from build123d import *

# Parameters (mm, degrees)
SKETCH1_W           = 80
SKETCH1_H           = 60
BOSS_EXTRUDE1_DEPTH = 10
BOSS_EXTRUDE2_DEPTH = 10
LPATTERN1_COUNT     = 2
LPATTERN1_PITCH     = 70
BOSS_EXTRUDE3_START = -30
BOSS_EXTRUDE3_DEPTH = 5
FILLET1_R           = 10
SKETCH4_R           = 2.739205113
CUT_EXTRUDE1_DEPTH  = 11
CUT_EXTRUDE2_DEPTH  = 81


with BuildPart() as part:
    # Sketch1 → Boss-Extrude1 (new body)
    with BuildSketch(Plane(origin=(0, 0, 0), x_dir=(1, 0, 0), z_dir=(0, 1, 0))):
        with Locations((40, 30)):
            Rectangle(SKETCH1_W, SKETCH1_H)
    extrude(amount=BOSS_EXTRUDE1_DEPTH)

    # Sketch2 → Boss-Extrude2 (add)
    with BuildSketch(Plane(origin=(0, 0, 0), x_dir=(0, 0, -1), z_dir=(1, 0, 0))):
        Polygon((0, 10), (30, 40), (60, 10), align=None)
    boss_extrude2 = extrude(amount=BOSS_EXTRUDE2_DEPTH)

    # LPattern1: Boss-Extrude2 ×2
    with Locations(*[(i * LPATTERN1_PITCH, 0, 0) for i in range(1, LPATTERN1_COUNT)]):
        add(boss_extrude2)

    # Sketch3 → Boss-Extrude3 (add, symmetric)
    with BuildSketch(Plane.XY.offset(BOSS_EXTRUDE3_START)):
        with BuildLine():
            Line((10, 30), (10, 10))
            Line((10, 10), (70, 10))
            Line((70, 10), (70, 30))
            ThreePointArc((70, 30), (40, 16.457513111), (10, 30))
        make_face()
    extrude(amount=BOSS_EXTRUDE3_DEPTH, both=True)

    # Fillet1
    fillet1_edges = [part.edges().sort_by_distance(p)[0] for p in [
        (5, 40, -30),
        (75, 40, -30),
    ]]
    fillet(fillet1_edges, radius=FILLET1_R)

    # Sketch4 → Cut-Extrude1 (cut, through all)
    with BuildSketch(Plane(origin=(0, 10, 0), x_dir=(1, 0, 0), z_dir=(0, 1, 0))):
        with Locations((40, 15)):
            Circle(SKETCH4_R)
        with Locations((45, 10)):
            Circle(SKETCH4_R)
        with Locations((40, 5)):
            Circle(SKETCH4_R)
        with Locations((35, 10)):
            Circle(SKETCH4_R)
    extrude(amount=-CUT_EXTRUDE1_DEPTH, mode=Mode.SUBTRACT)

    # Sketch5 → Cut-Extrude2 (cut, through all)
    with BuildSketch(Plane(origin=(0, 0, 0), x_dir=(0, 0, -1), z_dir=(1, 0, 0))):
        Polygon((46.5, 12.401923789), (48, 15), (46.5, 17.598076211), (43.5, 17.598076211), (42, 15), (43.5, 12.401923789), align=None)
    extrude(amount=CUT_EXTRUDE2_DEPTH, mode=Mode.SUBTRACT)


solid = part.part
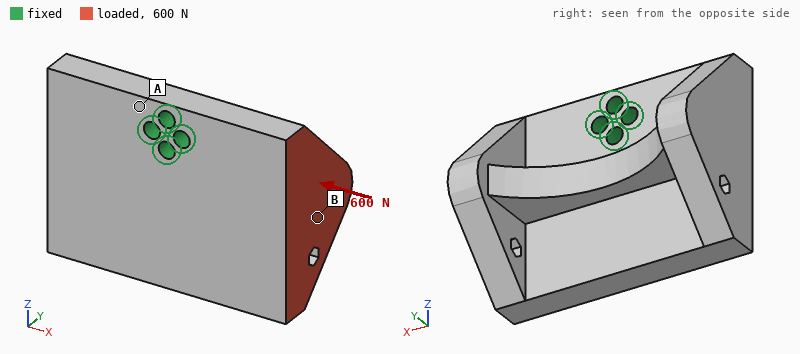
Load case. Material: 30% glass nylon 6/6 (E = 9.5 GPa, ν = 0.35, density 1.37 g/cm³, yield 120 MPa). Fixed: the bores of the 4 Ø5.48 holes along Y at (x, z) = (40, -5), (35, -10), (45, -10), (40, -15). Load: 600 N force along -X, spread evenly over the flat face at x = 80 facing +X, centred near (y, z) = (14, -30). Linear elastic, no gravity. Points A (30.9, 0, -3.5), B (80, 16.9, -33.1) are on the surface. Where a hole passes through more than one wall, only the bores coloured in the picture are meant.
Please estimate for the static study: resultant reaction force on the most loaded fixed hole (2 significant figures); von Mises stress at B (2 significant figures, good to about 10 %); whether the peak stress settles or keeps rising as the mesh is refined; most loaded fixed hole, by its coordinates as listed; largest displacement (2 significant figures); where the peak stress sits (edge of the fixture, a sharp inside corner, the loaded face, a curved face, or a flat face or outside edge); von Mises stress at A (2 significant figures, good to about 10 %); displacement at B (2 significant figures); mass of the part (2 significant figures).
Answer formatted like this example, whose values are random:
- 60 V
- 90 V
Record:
- 700 N
- 1.3 MPa
- keeps rising
- (40, -15)
- 95 µm
- edge of the fixture
- 4.4 MPa
- 73 µm
- 97 g
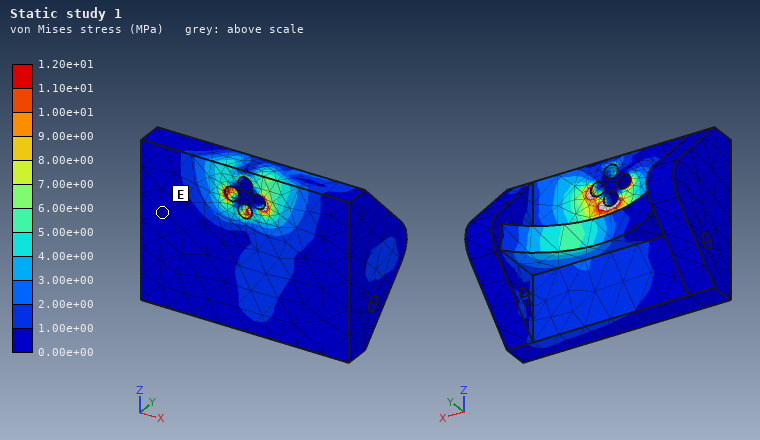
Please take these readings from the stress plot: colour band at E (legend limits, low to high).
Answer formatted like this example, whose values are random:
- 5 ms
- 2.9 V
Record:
- 0.00e+00 to 1.00e+00 MPa
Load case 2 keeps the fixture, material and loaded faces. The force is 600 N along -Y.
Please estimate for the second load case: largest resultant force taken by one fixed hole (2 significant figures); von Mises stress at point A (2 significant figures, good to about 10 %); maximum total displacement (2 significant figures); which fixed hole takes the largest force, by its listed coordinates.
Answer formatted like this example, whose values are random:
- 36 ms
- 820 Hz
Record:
- 700 N
- 8.7 MPa
- 0.42 mm
- (45, -10)
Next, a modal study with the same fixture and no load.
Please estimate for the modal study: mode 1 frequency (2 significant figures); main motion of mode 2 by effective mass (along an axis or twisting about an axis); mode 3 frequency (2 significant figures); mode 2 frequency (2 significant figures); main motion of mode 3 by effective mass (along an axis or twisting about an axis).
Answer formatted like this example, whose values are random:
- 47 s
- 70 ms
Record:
- 1300 Hz
- along Y
- 1900 Hz
- 1300 Hz
- along X
